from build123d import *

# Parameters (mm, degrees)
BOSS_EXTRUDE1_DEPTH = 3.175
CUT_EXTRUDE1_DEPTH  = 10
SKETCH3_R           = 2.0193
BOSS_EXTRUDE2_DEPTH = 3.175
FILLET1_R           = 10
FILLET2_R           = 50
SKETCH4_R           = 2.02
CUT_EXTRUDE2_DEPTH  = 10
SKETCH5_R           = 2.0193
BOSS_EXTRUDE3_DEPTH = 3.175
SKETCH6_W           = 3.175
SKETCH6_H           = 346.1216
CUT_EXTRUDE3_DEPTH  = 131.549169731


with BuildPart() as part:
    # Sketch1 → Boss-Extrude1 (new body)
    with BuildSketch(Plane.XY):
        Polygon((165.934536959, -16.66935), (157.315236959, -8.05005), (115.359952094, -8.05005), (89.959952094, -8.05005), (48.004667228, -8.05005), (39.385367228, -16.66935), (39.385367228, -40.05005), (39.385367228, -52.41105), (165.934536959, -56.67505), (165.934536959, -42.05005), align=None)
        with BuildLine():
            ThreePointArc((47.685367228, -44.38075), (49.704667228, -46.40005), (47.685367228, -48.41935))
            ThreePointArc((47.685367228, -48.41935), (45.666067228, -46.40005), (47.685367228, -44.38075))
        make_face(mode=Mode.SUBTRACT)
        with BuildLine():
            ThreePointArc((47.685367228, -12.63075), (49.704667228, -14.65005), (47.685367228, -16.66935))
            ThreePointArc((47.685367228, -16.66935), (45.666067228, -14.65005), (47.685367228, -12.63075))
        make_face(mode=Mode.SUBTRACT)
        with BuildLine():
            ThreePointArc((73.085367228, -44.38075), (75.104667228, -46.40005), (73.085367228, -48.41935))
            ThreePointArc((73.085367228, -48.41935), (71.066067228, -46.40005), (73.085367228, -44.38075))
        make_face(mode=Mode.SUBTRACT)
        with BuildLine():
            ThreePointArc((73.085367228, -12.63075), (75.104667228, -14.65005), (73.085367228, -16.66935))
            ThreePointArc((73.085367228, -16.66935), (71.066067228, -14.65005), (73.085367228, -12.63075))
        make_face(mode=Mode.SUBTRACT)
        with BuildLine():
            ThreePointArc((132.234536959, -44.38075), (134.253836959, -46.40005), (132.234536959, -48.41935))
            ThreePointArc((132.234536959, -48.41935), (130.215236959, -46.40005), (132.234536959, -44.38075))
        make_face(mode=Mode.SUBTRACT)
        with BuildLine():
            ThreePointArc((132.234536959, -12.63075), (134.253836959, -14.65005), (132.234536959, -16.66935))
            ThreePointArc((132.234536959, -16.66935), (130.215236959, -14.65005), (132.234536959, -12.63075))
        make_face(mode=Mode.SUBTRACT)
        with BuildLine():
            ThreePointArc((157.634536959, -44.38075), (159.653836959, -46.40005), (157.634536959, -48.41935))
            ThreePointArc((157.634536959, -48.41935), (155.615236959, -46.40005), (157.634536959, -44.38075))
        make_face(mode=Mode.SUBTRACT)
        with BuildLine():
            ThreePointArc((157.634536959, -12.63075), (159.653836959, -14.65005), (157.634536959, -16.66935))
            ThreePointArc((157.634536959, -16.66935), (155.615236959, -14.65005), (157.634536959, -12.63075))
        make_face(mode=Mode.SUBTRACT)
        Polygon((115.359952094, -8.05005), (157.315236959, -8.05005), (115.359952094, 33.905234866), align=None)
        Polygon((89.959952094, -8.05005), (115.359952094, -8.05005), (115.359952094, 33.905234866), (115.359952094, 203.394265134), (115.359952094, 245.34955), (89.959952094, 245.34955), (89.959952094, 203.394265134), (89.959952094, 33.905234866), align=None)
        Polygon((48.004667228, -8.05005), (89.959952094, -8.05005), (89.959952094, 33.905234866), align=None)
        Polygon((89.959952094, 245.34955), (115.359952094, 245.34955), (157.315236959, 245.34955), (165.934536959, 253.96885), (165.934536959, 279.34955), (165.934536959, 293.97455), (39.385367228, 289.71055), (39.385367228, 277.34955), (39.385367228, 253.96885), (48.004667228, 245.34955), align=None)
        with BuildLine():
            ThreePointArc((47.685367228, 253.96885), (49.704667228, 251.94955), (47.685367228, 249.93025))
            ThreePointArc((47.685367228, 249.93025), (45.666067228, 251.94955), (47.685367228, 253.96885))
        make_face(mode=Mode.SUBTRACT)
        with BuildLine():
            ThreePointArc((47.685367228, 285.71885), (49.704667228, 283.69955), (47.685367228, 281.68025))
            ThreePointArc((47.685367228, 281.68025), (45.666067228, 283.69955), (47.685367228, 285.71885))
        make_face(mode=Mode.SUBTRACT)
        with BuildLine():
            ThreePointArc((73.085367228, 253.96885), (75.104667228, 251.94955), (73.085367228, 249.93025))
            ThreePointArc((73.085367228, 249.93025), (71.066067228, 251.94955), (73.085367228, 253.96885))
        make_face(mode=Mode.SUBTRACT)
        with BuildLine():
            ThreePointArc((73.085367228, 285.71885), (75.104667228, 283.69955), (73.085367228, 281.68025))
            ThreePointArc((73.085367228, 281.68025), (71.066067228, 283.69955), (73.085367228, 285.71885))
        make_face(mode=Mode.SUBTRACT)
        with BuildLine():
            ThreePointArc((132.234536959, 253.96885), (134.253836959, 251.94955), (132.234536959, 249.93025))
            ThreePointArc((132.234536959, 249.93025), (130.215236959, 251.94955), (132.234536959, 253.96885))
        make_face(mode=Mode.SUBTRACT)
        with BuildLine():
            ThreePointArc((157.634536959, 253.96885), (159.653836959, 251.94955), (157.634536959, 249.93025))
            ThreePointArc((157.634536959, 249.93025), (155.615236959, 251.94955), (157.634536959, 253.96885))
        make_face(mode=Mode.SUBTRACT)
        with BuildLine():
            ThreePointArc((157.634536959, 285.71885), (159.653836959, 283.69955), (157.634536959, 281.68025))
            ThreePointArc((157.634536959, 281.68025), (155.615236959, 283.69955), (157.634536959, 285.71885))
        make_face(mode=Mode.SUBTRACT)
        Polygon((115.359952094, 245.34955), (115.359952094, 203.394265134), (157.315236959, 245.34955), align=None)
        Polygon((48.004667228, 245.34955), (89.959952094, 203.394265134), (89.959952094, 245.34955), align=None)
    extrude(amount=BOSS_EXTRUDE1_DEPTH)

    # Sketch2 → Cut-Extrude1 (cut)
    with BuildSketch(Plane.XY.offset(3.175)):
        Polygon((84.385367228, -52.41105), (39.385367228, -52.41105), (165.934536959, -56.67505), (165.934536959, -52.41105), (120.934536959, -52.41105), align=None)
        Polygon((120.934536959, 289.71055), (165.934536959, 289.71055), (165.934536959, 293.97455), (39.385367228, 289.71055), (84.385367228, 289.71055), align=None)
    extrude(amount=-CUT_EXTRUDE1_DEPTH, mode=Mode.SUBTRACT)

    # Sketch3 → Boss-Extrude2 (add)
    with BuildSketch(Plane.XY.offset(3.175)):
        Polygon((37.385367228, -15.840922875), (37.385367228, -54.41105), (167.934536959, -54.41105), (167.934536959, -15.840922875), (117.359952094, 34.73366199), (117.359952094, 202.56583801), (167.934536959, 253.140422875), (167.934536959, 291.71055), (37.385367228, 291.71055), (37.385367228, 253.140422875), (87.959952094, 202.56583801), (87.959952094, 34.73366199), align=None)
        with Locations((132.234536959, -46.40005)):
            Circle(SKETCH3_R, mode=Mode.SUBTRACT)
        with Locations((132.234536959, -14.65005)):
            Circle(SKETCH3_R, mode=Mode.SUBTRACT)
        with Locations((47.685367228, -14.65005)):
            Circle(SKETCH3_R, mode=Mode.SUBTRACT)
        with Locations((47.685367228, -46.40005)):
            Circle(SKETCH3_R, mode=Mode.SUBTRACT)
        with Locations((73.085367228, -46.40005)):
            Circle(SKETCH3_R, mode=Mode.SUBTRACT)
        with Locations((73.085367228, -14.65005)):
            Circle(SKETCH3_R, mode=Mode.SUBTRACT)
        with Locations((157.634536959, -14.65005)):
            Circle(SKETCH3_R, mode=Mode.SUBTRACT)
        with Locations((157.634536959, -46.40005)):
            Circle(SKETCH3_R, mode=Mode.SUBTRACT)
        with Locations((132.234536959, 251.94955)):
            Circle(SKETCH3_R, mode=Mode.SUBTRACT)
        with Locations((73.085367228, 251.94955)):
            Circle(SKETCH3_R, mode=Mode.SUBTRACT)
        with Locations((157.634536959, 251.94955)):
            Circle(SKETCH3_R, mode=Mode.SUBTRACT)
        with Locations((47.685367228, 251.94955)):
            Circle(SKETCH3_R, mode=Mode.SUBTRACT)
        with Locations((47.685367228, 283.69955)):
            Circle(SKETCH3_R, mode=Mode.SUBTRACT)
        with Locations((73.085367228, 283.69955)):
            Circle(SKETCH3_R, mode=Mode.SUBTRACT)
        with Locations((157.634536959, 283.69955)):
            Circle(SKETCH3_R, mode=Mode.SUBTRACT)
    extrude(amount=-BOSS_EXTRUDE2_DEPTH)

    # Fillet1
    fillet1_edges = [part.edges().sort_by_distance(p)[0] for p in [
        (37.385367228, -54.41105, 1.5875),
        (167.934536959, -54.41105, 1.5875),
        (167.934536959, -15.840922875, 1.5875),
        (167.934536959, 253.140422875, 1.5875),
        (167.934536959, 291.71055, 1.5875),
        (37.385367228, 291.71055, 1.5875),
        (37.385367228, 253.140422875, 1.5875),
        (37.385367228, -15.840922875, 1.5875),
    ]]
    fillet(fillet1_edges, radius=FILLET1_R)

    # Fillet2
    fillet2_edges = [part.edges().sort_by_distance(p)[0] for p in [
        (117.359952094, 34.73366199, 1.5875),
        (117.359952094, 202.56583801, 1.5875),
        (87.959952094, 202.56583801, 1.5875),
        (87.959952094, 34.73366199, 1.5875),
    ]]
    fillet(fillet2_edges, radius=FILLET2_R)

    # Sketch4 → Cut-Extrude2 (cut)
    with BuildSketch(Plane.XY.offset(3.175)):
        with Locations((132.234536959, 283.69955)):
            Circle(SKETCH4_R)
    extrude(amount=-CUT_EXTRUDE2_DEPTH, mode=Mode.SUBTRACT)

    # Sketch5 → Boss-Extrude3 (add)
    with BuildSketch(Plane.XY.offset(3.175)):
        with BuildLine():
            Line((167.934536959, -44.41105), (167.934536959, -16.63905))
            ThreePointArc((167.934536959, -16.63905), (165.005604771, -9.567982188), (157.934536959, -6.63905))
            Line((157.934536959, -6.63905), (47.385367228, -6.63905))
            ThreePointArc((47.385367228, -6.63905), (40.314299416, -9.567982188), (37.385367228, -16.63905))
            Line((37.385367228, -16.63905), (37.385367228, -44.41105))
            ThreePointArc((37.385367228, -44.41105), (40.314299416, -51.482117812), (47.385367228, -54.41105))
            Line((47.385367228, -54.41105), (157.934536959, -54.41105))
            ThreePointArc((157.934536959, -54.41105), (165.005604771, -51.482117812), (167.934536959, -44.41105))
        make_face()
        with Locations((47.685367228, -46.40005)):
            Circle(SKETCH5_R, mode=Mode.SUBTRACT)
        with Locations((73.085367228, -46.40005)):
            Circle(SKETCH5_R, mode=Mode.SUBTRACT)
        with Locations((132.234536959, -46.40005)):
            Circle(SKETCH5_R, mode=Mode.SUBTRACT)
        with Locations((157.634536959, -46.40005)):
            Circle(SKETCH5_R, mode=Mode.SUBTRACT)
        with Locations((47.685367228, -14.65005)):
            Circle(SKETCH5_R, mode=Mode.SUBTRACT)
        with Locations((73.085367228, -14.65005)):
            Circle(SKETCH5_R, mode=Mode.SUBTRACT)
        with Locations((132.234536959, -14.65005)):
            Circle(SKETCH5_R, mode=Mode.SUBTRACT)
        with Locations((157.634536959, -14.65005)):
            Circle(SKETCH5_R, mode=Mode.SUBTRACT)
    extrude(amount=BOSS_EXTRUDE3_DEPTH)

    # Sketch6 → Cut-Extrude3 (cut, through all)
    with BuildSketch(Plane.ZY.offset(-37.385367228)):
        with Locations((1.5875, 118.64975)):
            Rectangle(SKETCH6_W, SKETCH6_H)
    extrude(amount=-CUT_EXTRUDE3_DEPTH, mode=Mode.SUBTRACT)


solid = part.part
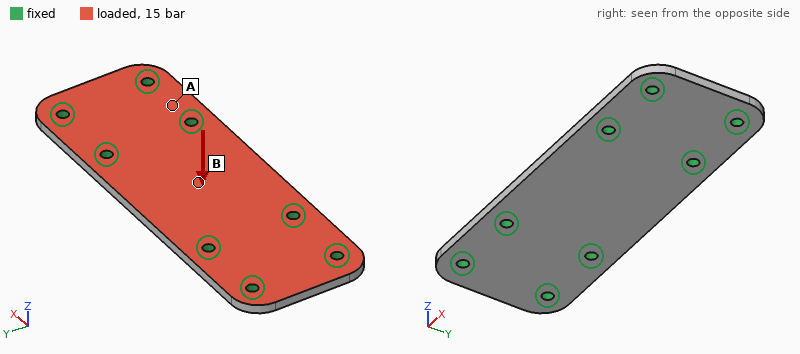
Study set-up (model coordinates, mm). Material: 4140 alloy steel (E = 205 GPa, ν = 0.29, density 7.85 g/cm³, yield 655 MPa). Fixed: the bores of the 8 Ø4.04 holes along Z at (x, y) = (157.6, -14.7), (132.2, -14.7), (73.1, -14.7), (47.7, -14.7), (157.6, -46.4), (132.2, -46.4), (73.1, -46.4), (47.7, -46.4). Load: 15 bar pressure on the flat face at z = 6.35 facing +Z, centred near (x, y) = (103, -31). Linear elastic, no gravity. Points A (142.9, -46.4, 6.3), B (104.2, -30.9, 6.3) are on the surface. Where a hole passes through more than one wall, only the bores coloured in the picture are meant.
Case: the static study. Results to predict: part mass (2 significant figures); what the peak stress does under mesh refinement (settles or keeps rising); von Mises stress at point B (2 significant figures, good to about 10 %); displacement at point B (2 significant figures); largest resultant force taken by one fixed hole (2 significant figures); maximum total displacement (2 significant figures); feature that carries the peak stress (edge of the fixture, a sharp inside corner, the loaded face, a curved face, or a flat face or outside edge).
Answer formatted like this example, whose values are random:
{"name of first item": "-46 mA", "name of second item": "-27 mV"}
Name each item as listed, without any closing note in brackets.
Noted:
{"part mass": "150 g", "what the peak stress does under mesh refinement": "keeps rising", "von Mises stress at point B": "110 MPa", "displacement at point B": "93 µm", "largest resultant force taken by one fixed hole": "1.6 kN", "maximum total displacement": "93 µm", "feature that carries the peak stress": "edge of the fixture"}
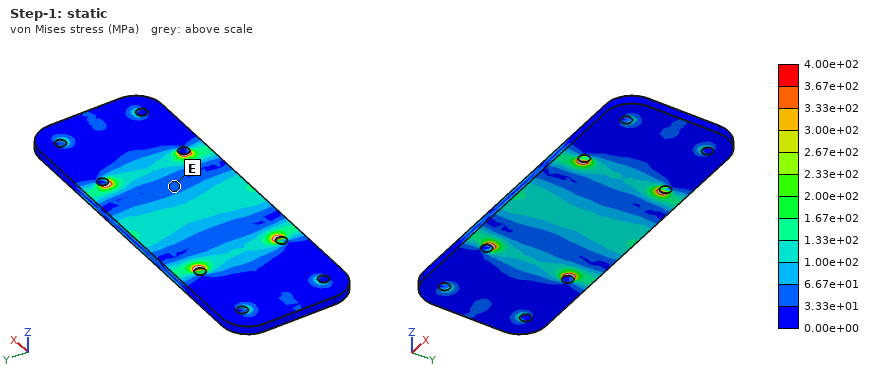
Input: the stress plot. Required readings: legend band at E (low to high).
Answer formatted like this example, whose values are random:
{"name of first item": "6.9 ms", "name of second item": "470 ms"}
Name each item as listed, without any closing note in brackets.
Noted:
{"legend band at E": "3.33e+01 to 6.67e+01 MPa"}
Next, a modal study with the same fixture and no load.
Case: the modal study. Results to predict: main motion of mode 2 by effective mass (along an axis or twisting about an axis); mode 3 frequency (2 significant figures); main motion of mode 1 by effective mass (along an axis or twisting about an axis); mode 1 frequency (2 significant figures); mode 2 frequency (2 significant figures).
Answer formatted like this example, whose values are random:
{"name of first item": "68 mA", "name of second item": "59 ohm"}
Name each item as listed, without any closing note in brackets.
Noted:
{"main motion of mode 2 by effective mass": "twisting about X", "mode 3 frequency": "11 kHz", "main motion of mode 1 by effective mass": "along Z", "mode 1 frequency": "4600 Hz", "mode 2 frequency": "6200 Hz"}
